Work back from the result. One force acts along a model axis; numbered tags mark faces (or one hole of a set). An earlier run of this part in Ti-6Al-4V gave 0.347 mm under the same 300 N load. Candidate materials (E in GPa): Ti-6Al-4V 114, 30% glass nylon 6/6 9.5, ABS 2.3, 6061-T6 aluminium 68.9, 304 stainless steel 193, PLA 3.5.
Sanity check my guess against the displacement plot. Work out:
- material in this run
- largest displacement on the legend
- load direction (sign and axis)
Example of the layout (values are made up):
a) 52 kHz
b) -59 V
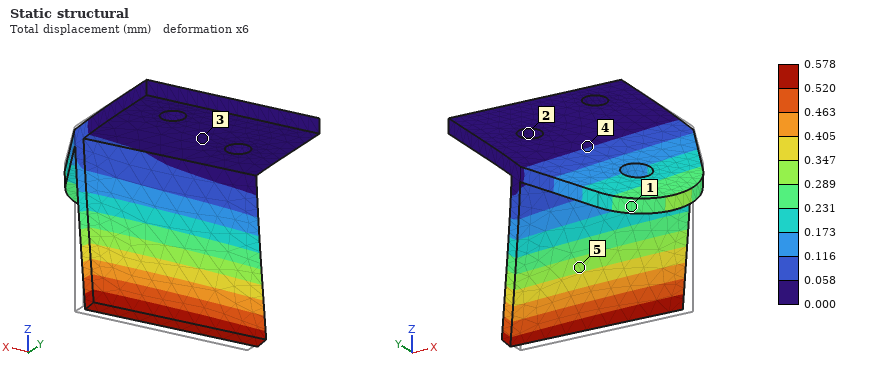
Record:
a) 6061-T6 aluminium
b) 0.578 mm
c) +Y
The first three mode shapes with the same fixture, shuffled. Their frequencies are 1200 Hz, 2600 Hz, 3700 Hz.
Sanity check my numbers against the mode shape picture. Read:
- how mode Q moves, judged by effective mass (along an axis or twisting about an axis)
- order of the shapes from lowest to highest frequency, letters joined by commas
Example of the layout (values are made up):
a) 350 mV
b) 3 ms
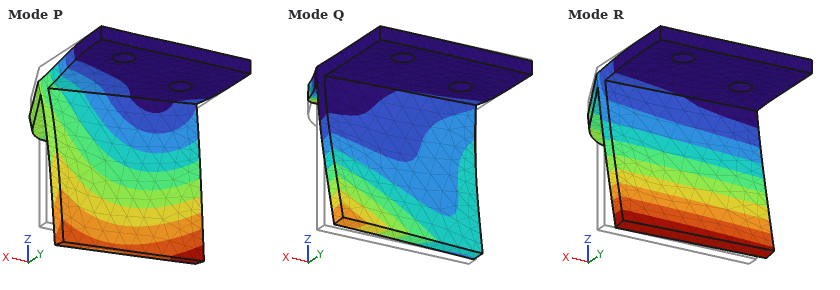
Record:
a) along Z
b) R, P, Q
